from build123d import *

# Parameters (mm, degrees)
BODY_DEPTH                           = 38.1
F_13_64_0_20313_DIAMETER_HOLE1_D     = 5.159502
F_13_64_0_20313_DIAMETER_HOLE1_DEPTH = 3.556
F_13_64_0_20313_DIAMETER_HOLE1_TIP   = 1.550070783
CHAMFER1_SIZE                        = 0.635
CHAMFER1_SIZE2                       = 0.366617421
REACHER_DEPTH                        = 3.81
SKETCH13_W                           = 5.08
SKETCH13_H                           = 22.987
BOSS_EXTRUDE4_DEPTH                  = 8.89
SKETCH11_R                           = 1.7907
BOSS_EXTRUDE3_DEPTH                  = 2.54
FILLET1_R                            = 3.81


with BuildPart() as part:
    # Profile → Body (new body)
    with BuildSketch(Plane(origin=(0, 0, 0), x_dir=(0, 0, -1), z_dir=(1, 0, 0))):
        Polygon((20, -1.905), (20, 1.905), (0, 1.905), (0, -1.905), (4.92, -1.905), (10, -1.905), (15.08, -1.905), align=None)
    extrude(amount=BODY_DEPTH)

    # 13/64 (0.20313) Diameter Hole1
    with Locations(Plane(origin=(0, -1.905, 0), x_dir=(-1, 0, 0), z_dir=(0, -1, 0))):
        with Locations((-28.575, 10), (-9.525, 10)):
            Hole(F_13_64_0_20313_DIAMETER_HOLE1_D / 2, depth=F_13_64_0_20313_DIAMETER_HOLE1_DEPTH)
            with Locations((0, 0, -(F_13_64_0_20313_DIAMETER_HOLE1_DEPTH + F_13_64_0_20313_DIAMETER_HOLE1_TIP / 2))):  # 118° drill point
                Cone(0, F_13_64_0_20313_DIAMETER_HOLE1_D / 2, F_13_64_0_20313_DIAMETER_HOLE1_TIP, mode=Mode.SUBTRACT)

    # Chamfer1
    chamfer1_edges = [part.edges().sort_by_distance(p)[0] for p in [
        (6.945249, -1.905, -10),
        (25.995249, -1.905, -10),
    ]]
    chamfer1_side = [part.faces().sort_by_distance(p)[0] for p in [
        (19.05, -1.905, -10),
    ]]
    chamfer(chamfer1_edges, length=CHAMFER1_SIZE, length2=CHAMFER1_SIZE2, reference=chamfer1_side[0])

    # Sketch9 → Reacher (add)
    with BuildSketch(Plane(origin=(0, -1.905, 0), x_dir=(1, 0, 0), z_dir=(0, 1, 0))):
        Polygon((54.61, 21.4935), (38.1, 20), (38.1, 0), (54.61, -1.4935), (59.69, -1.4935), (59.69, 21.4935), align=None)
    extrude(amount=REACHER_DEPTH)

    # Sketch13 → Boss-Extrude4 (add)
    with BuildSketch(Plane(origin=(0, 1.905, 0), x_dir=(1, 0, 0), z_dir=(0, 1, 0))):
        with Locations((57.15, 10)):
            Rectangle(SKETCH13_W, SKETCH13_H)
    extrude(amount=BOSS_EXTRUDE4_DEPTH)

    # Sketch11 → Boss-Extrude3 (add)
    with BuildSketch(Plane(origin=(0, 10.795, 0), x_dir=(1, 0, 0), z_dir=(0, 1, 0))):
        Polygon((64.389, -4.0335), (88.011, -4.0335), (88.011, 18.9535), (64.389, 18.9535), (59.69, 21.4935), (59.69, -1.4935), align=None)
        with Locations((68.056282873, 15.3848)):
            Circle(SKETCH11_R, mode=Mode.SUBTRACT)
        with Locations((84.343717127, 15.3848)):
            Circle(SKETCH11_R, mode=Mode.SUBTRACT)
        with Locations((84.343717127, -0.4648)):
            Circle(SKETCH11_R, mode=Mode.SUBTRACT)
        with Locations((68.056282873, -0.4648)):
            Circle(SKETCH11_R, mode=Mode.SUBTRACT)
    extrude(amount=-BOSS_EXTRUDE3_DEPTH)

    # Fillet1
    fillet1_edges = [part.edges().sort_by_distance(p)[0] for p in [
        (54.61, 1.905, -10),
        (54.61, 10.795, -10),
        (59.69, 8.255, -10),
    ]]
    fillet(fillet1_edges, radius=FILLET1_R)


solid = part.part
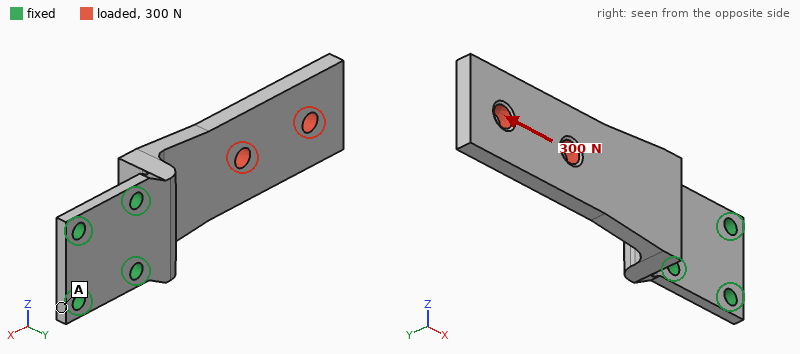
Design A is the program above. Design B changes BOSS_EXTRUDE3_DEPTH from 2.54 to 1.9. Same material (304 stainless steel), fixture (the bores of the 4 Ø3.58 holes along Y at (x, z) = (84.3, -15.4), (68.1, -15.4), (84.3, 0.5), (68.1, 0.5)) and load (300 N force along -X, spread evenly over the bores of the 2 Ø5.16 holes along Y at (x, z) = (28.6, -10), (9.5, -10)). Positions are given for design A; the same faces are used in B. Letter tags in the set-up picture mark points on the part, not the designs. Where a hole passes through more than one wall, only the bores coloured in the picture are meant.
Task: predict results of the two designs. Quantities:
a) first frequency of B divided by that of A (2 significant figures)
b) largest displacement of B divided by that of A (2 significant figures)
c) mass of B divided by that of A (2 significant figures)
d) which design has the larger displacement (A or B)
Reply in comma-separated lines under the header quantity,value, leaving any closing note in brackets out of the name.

quantity,value
first frequency of B divided by that of A,0.73
largest displacement of B divided by that of A,2.2
mass of B divided by that of A,0.95
which design has the larger displacement,B
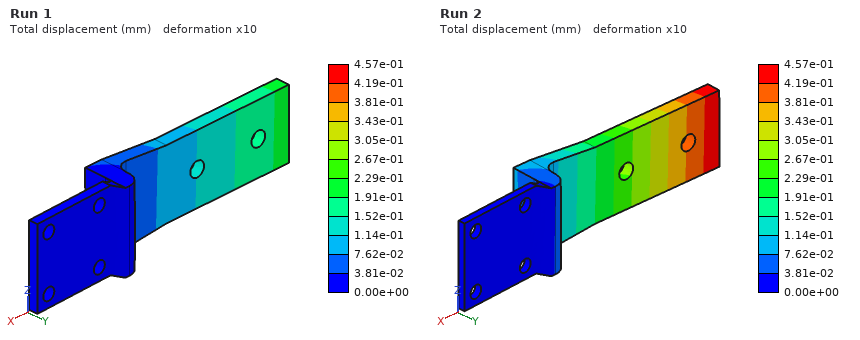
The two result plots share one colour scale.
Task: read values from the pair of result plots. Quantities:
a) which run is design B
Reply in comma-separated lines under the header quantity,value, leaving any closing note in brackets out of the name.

quantity,value
which run is design B,Run 2
